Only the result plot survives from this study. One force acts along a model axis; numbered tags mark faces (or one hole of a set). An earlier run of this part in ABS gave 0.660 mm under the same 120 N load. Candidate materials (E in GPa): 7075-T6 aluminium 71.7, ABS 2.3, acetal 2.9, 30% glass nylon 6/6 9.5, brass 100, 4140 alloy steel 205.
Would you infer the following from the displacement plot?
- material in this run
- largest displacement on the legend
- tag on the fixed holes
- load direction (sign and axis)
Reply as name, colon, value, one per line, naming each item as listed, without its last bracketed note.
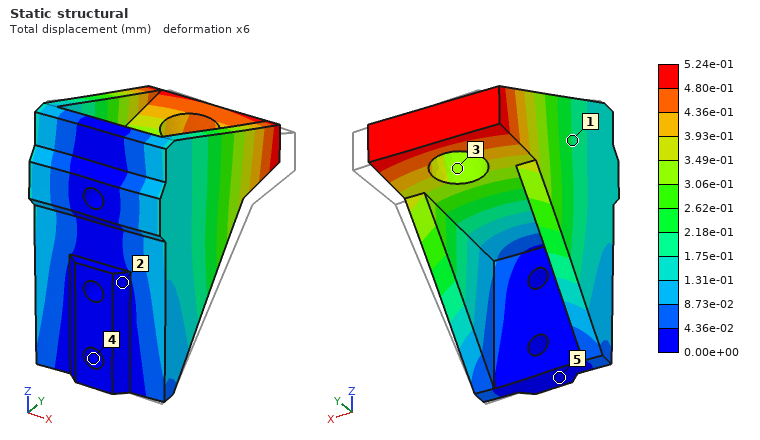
material in this run: acetal
largest displacement on the legend: 5.24e-01 mm
tag on the fixed holes: 4
load direction: -X
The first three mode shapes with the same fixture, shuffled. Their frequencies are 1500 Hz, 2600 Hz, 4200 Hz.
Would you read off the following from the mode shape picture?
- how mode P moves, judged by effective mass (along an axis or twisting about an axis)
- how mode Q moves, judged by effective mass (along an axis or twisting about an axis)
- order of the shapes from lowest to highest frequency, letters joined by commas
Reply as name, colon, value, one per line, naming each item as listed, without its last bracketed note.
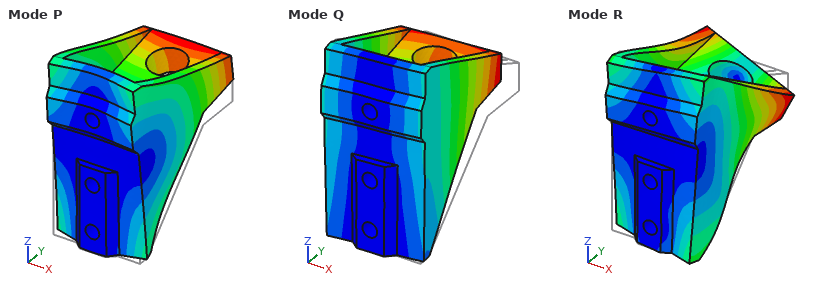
how mode P moves, judged by effective mass: along Z
how mode Q moves, judged by effective mass: along X
order of the shapes from lowest to highest frequency, letters joined by commas: Q, P, R
